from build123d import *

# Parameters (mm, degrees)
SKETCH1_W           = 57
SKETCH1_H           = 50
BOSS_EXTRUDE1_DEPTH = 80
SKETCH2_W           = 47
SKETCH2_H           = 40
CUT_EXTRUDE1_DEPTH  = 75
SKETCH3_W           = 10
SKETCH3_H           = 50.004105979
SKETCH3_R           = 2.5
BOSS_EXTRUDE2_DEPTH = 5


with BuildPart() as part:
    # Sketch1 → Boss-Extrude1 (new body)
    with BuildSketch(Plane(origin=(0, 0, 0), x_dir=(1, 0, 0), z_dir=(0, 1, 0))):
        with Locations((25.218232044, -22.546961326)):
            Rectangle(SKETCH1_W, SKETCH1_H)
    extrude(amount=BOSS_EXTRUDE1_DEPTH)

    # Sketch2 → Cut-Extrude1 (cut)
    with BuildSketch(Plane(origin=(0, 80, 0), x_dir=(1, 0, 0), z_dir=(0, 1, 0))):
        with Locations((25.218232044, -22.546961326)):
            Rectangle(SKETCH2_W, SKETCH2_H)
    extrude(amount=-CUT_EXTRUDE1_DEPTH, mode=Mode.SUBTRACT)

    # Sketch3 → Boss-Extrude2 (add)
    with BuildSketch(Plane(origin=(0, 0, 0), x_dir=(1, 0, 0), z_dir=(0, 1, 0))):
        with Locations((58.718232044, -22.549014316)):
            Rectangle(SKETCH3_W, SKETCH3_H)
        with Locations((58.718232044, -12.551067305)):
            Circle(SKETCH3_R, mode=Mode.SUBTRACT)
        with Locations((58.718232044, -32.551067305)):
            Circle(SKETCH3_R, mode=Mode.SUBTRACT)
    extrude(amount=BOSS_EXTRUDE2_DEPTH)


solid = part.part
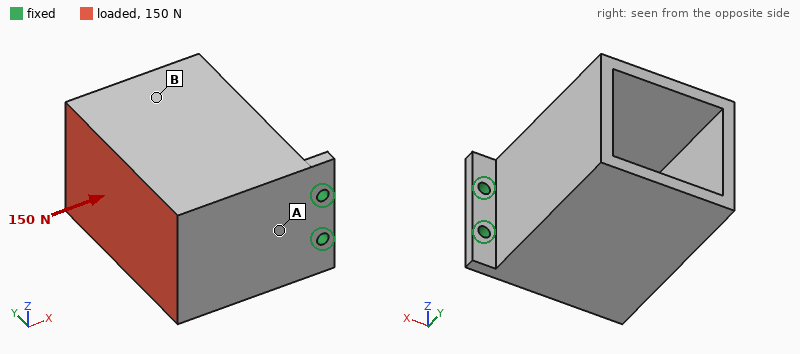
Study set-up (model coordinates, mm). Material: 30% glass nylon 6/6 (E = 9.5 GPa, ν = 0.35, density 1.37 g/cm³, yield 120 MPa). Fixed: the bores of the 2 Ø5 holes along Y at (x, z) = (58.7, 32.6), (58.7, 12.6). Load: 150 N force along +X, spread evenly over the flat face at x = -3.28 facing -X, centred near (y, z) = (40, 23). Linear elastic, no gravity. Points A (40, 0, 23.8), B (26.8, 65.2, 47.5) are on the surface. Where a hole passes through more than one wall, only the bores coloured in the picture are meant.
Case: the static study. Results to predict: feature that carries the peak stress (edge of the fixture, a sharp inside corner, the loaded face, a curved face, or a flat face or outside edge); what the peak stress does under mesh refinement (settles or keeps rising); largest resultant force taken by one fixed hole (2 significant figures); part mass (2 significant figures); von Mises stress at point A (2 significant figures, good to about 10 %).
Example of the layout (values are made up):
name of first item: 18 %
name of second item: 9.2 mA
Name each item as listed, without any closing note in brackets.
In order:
feature that carries the peak stress: edge of the fixture
what the peak stress does under mesh refinement: keeps rising
largest resultant force taken by one fixed hole: 79 N
part mass: 120 g
von Mises stress at point A: 4.5 MPa
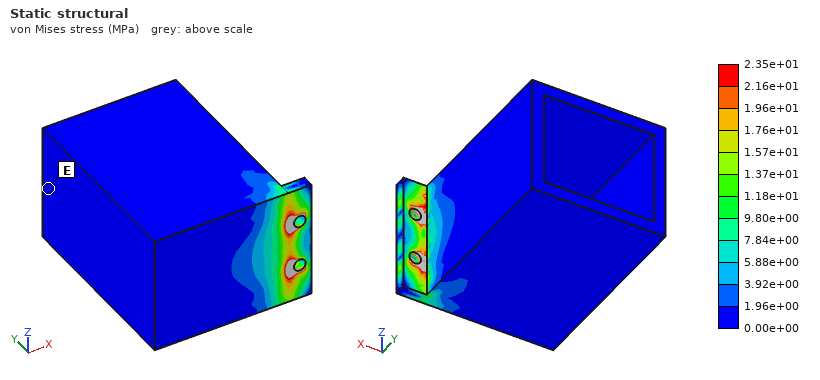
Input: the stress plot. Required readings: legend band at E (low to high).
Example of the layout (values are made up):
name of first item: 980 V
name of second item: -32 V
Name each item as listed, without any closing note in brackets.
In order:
legend band at E: 0.00e+00 to 1.96e+00 MPa
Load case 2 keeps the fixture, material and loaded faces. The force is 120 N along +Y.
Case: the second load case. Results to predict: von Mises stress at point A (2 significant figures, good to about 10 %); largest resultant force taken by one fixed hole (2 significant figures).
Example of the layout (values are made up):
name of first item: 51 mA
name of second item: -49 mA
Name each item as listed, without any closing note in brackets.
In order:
von Mises stress at point A: 5.9 MPa
largest resultant force taken by one fixed hole: 61 N
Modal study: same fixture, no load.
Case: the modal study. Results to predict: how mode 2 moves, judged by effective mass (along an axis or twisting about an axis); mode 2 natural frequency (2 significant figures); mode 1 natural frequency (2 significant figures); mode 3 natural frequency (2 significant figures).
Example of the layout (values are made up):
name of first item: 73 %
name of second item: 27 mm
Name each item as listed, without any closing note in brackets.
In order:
how mode 2 moves, judged by effective mass: along Z
mode 2 natural frequency: 600 Hz
mode 1 natural frequency: 190 Hz
mode 3 natural frequency: 1300 Hz
